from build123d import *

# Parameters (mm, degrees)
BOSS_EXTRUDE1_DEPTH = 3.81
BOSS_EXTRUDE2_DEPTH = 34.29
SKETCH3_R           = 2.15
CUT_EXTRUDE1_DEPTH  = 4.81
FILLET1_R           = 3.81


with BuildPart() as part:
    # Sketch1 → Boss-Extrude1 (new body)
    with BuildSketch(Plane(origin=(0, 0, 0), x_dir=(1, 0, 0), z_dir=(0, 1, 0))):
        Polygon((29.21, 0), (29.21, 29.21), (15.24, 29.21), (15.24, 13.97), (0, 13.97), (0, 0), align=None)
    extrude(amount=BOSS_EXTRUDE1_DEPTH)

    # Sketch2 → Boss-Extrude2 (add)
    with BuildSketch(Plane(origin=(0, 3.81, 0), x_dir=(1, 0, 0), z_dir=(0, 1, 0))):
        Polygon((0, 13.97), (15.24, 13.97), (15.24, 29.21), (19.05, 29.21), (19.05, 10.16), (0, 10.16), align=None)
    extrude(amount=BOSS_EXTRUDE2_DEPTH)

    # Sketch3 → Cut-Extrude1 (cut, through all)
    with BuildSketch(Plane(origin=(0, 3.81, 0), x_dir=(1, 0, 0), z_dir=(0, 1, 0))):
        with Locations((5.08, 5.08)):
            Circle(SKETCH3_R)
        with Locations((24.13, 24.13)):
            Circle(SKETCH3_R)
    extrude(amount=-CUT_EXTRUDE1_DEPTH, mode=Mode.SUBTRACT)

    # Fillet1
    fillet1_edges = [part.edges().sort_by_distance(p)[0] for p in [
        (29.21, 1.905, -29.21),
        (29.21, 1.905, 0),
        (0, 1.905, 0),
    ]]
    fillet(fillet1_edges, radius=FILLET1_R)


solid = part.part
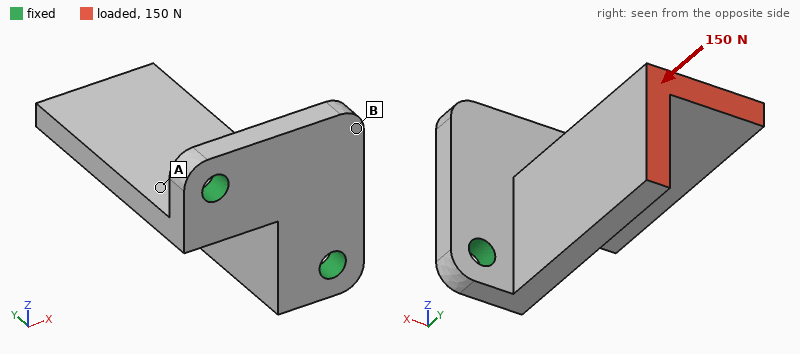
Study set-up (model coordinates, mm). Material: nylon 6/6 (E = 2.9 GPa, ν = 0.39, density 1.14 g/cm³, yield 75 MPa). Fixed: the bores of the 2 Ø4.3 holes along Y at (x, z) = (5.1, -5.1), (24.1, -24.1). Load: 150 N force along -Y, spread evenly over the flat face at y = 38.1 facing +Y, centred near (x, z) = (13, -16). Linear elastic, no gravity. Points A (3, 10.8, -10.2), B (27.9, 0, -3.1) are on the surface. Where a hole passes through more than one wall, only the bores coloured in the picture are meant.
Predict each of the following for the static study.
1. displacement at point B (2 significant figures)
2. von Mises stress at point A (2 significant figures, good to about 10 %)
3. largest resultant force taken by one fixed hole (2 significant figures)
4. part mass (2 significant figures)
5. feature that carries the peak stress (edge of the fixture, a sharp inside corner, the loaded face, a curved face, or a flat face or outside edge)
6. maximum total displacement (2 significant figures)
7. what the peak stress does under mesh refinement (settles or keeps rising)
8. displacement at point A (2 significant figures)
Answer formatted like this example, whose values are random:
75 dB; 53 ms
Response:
11 µm; 2.4 MPa; 78 N; 7.6 g; edge of the fixture; 43 µm; keeps rising; 31 µm
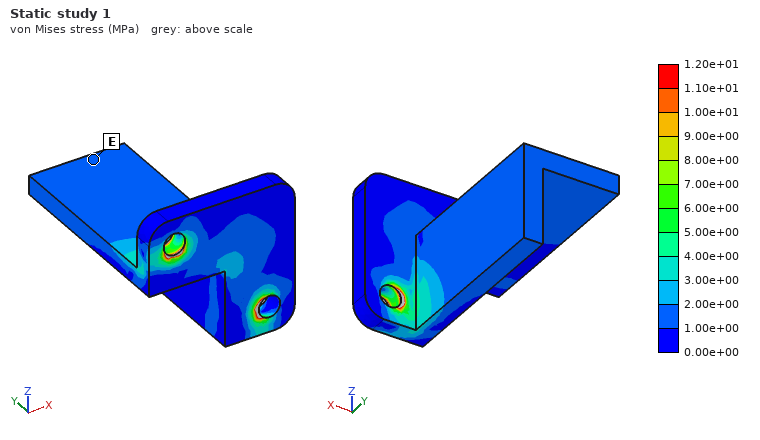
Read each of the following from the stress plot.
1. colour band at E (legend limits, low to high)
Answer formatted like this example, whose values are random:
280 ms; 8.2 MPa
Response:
1.00e+00 to 2.00e+00 MPa
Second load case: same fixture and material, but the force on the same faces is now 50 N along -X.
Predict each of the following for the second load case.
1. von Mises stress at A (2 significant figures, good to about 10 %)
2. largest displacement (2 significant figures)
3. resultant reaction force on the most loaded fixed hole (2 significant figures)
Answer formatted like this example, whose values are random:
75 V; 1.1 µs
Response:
4.8 MPa; 0.61 mm; 64 N
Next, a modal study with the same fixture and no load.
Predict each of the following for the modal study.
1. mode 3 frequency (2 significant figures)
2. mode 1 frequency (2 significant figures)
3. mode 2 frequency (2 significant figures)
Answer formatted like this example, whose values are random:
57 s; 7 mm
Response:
2400 Hz; 1000 Hz; 1800 Hz
